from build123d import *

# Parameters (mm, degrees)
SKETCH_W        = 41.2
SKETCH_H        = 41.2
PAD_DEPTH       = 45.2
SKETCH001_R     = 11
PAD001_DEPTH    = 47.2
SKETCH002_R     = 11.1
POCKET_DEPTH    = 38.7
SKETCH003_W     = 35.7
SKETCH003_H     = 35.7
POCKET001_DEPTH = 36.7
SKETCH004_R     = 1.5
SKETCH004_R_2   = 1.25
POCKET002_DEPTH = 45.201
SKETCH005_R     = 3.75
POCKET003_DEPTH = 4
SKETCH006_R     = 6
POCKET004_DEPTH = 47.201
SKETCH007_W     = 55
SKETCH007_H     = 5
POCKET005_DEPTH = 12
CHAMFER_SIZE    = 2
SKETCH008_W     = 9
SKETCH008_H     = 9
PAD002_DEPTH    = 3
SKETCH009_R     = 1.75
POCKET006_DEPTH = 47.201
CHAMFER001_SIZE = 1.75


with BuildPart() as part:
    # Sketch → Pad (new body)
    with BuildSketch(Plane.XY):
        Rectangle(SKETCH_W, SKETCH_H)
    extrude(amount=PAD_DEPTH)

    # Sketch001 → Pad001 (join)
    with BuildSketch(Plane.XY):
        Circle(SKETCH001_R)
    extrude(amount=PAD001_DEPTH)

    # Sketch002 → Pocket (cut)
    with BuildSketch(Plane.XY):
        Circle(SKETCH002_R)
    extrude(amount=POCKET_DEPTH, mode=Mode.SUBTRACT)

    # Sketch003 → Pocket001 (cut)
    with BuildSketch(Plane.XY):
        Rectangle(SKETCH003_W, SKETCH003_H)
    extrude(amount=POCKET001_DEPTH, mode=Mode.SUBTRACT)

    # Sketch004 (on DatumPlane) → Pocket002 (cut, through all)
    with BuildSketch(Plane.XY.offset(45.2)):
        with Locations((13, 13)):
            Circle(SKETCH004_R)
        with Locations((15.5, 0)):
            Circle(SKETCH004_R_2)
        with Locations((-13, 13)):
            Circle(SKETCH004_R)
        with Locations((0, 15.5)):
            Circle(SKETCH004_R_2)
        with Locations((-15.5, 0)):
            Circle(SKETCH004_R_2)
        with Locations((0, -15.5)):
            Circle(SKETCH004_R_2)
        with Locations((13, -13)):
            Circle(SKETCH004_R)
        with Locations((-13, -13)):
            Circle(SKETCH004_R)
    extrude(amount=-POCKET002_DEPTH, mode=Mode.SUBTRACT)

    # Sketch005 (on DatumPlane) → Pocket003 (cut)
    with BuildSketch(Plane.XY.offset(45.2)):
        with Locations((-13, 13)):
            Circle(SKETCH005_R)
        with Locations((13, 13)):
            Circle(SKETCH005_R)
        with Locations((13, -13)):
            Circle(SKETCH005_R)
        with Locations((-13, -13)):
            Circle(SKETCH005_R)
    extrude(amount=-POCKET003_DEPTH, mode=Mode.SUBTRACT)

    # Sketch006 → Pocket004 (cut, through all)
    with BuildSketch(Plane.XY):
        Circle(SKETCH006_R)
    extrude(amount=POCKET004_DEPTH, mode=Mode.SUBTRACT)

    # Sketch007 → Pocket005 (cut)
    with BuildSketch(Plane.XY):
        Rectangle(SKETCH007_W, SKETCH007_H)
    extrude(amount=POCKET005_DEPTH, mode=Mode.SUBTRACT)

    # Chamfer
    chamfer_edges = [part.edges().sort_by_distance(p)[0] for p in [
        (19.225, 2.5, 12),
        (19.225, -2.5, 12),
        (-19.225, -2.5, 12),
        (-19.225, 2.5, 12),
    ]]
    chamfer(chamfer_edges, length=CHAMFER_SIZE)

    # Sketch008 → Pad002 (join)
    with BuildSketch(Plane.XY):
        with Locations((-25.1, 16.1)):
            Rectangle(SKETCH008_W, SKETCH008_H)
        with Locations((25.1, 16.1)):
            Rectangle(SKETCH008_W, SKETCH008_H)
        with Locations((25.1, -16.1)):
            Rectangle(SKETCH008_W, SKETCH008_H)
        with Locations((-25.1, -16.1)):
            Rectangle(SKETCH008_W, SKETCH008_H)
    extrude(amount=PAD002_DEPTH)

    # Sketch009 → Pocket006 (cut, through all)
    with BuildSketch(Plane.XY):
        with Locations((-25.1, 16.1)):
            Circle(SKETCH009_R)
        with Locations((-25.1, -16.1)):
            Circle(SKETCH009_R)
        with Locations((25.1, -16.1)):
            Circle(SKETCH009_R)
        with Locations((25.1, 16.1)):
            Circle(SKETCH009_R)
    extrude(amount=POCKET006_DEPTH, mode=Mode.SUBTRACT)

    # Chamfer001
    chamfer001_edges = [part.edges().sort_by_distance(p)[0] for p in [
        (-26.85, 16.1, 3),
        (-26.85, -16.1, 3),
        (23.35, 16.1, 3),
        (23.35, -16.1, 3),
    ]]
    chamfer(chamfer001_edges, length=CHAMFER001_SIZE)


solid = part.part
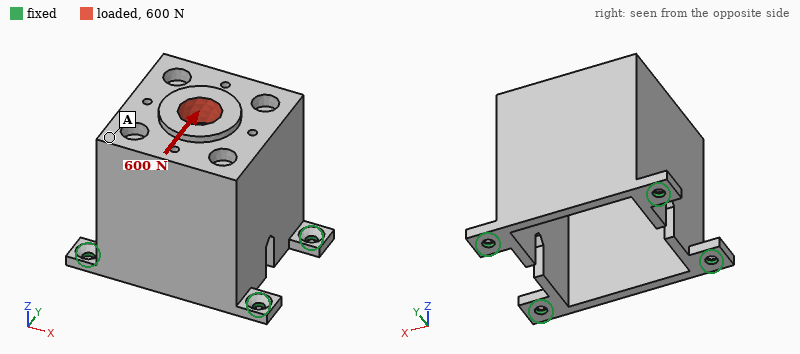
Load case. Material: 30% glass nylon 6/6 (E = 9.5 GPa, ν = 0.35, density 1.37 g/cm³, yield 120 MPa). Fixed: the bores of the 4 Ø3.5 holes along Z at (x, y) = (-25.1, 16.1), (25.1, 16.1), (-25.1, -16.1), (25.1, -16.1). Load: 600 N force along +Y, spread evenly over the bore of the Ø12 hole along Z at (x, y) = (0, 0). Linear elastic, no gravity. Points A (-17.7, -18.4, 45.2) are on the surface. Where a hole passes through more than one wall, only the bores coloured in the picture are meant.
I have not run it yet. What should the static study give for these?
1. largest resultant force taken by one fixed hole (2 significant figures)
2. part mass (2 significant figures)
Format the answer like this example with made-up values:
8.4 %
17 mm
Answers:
430 N
39 g
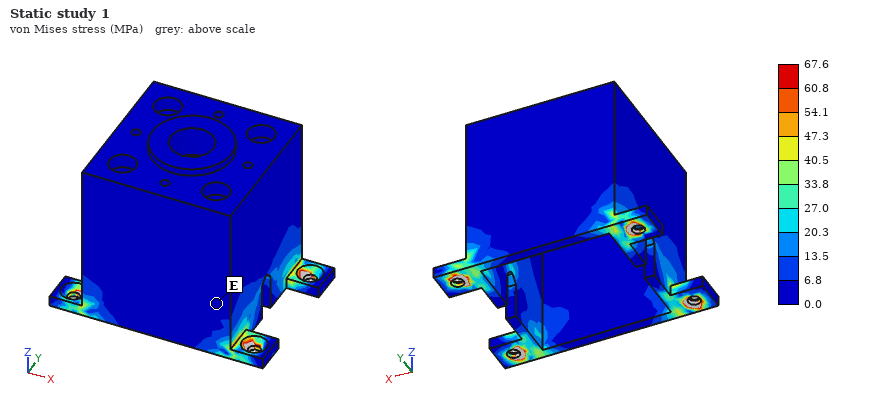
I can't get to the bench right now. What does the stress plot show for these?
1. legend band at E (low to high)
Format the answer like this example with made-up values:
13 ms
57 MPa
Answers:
0.0 to 6.8 MPa
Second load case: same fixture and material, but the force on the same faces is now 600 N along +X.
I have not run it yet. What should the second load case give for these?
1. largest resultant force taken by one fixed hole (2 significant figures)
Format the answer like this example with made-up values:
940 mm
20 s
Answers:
320 N
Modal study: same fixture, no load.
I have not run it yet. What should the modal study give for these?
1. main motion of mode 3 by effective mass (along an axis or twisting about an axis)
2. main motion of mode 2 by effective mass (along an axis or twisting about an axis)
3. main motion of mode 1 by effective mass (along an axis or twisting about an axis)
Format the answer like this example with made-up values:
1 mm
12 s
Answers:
along Z
along X
along Y
